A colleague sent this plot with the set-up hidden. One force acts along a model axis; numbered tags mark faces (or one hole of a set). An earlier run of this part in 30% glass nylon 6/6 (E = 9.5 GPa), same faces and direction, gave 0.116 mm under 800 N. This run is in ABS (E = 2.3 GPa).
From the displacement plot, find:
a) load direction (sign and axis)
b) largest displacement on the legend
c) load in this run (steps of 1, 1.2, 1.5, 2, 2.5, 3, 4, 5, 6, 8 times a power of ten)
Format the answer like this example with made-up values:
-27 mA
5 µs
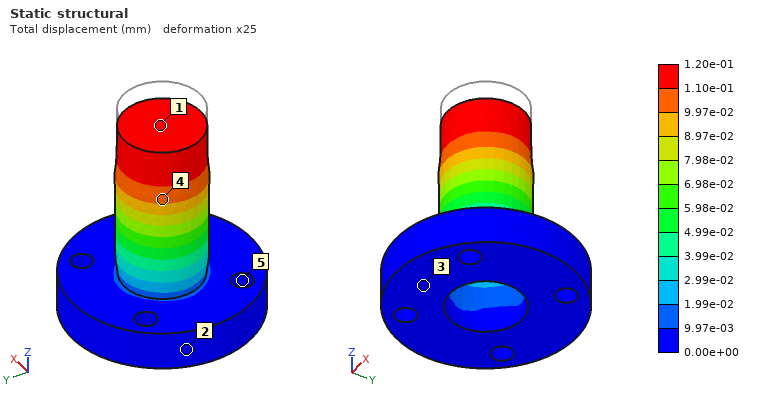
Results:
-Z
1.20e-01 mm
200 N
